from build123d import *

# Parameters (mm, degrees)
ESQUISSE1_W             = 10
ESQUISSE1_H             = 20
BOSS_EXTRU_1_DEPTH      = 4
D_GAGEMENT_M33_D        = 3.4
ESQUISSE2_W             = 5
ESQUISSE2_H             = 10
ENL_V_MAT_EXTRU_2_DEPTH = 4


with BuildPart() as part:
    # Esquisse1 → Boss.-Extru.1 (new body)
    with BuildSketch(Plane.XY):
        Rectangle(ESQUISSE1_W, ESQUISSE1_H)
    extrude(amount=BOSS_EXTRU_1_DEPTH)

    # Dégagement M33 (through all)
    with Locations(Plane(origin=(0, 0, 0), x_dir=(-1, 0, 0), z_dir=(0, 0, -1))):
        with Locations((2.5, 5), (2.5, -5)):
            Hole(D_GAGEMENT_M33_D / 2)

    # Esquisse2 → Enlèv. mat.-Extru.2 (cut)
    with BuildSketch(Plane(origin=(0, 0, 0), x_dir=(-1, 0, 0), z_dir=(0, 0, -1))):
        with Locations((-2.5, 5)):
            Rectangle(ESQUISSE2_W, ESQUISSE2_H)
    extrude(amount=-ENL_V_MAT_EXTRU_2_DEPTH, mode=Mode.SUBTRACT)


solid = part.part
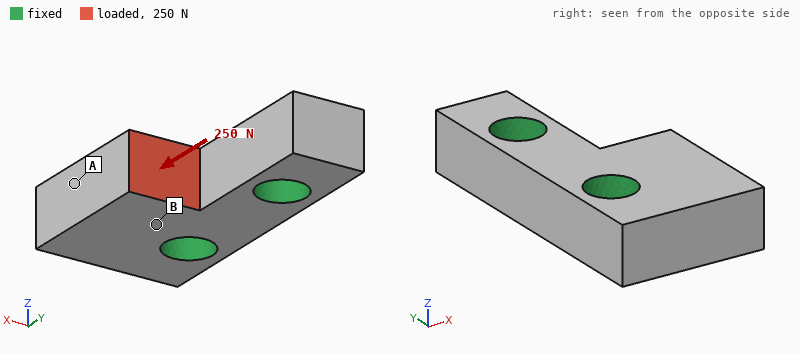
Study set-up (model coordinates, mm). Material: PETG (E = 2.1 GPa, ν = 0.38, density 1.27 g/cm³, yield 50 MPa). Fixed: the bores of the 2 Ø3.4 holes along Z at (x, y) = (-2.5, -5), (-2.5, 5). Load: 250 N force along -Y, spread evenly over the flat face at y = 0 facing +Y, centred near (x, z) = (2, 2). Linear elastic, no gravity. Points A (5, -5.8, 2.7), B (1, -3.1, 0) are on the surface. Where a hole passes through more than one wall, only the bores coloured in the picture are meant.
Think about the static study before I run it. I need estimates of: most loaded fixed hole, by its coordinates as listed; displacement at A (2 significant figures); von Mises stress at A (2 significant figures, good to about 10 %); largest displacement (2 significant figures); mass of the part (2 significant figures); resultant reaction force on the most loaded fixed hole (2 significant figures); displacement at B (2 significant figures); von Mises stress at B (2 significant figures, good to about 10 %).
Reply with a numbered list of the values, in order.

1. (-2.5, -5)
2. 0.075 mm
3. 3.9 MPa
4. 0.11 mm
5. 0.67 g
6. 200 N
7. 0.035 mm
8. 14 MPa
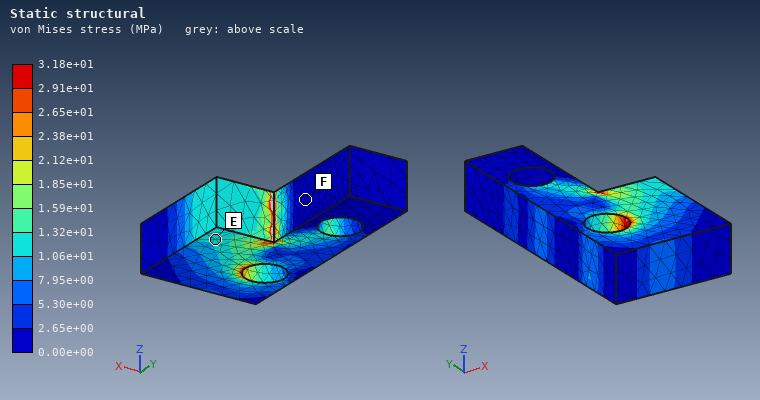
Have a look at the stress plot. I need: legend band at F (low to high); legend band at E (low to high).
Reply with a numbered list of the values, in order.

1. 0.00e+00 to 2.65e+00 MPa
2. 1.06e+01 to 1.32e+01 MPa
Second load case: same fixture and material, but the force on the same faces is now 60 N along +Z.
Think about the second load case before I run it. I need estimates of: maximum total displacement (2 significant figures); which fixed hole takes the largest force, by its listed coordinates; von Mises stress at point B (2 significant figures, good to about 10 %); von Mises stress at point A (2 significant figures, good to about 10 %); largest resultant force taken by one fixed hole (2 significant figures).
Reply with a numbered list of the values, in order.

1. 99 µm
2. (-2.5, -5)
3. 10 MPa
4. 1.9 MPa
5. 43 N
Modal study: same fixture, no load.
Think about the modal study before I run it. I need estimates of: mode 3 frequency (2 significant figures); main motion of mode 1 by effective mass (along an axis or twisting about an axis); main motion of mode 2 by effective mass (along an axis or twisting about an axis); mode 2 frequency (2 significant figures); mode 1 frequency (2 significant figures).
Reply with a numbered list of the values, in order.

1. 19 kHz
2. along Z
3. along Y
4. 18 kHz
5. 15 kHz
